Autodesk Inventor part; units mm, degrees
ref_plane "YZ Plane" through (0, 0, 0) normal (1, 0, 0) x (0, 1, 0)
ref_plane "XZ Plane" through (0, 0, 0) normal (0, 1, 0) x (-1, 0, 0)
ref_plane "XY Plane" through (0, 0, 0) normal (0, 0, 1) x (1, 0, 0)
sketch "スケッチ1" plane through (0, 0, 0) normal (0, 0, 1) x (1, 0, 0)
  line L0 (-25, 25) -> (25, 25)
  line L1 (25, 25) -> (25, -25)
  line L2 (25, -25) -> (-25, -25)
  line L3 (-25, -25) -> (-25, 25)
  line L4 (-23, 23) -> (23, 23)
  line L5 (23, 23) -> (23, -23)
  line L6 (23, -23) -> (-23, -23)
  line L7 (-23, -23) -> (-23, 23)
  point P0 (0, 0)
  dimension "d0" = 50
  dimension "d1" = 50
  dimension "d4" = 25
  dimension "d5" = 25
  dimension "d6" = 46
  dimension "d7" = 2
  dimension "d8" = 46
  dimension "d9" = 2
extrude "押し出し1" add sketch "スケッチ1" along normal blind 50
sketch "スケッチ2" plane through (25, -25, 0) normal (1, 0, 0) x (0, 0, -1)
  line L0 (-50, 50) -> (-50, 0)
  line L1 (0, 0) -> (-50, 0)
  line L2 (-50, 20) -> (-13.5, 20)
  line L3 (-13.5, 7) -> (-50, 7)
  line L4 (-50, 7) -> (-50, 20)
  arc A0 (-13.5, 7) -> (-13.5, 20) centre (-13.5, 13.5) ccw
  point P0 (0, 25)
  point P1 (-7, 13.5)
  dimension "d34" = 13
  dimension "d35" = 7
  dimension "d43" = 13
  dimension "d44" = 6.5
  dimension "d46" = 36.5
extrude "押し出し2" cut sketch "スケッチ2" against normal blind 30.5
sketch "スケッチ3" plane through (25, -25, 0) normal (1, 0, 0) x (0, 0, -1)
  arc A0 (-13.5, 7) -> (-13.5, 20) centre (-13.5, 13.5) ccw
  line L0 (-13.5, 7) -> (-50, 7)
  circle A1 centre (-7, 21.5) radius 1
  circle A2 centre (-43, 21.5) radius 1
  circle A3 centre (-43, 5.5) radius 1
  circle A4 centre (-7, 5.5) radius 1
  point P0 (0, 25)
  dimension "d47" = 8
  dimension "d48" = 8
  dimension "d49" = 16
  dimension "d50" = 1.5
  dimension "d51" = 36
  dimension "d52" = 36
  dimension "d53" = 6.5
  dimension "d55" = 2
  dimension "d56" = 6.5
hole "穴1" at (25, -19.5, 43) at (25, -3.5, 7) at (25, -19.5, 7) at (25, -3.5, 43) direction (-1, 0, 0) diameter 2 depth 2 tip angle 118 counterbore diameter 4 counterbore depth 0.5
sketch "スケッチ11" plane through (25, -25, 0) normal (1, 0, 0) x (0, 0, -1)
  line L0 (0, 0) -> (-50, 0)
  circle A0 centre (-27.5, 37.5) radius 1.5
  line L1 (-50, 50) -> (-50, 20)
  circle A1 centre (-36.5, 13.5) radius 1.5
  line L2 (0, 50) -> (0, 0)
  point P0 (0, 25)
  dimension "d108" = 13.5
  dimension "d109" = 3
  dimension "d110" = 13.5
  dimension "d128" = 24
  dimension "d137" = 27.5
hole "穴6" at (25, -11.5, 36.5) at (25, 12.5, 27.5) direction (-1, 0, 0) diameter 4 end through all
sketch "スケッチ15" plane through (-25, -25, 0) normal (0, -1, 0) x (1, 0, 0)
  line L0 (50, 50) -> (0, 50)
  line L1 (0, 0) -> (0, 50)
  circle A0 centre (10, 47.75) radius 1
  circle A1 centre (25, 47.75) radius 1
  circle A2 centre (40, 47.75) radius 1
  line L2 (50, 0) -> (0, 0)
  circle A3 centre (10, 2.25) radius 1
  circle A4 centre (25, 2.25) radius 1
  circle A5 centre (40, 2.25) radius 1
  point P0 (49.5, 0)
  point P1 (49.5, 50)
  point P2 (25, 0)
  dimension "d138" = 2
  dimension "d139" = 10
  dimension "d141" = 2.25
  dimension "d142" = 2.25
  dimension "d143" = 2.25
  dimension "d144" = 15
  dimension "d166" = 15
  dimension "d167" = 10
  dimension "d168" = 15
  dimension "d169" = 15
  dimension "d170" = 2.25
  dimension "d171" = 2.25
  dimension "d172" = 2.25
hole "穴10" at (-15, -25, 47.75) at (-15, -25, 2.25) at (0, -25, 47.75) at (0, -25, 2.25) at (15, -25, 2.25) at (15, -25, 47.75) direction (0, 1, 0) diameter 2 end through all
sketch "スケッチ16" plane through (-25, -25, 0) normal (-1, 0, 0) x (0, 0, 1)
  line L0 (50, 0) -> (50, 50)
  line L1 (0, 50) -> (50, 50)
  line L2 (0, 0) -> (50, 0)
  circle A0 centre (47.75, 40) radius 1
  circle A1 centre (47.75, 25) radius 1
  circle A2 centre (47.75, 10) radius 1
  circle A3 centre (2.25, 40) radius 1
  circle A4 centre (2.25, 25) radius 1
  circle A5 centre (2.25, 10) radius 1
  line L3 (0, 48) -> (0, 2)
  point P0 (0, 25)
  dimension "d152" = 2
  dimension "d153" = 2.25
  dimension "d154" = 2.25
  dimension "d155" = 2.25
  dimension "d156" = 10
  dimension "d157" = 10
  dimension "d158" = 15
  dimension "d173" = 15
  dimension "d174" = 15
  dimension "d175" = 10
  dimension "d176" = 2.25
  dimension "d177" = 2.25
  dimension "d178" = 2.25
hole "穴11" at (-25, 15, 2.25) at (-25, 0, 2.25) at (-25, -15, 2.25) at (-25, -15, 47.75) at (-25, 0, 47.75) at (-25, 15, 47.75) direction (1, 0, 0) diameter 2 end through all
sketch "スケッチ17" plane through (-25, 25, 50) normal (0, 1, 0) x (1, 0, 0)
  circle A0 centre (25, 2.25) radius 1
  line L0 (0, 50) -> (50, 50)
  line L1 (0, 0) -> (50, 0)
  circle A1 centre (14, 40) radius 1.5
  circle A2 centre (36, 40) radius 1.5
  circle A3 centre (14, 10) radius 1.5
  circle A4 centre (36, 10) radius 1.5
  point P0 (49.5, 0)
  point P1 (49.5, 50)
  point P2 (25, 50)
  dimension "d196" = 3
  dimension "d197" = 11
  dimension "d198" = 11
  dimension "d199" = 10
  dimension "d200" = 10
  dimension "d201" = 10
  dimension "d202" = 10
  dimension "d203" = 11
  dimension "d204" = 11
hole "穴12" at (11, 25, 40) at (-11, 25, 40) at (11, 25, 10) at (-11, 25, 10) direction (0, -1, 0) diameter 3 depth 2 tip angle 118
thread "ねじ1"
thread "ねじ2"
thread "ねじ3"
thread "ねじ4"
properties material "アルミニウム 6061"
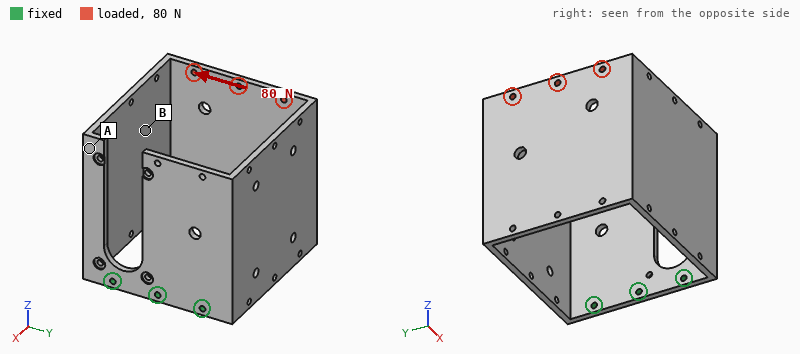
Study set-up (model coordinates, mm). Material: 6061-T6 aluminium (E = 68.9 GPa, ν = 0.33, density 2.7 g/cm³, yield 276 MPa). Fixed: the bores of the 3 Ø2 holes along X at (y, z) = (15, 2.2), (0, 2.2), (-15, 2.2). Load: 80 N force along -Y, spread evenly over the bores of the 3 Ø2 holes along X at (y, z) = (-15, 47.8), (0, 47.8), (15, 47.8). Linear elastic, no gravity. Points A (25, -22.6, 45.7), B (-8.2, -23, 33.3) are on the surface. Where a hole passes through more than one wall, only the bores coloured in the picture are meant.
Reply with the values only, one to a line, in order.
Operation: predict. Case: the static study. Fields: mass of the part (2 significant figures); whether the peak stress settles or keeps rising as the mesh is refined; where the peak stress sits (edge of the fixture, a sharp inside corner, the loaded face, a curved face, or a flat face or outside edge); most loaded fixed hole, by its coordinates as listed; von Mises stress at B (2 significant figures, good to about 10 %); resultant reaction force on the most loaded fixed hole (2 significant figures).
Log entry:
48 g
keeps rising
edge of the fixture
(15, 2.2)
19 MPa
150 N
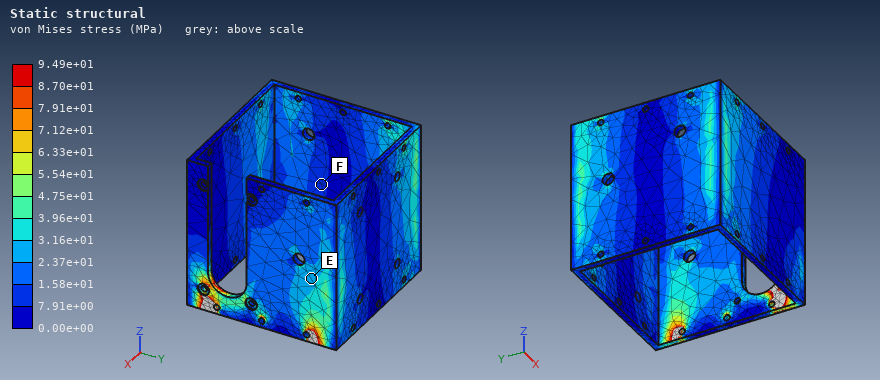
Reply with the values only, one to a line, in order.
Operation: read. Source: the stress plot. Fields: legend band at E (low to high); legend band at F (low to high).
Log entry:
2.37e+01 to 3.16e+01 MPa
7.91e+00 to 1.58e+01 MPa
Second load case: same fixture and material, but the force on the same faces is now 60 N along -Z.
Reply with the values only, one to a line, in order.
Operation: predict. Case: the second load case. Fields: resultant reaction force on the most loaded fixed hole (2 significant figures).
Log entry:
55 N
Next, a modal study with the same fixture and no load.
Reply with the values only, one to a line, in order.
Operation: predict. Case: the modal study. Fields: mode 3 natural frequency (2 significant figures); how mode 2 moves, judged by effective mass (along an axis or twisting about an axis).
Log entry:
730 Hz
along Y
